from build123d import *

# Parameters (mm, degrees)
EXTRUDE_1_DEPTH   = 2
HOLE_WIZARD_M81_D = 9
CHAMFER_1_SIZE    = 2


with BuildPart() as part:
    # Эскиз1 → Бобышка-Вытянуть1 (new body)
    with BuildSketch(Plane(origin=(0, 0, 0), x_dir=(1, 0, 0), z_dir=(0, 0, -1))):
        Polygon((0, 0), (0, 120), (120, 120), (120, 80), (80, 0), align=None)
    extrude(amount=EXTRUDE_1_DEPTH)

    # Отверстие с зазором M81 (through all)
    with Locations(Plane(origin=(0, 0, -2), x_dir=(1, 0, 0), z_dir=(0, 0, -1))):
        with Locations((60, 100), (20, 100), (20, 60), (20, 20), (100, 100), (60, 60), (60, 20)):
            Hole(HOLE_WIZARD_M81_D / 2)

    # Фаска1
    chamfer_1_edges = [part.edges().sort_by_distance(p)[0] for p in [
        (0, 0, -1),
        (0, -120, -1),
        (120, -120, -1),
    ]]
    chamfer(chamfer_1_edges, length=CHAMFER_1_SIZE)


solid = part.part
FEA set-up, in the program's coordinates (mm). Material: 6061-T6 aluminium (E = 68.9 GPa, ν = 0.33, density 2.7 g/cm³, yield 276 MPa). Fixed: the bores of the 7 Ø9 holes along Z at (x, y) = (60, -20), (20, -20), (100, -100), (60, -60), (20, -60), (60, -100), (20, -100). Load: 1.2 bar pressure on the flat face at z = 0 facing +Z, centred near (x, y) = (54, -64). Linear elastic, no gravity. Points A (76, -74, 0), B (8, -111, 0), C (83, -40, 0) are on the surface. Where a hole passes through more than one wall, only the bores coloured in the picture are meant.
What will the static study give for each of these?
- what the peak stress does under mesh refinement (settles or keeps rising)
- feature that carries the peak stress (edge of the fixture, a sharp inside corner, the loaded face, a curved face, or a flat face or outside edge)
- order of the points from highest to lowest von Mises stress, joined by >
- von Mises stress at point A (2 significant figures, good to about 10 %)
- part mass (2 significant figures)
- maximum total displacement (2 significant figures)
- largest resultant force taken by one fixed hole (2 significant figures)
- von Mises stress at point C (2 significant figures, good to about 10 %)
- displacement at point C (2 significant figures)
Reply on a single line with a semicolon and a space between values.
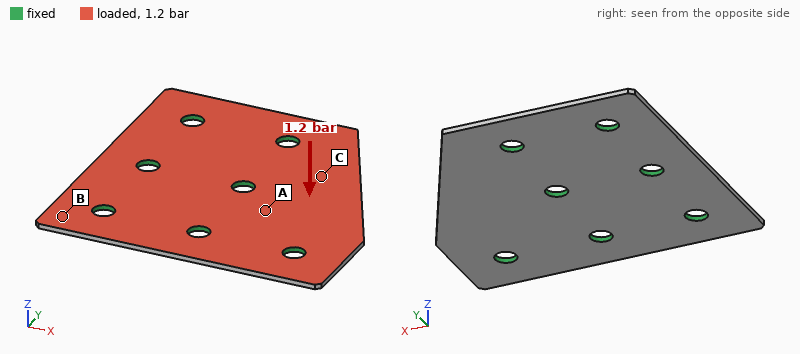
keeps rising; edge of the fixture; A > C > B; 30 MPa; 67 g; 0.43 mm; 260 N; 20 MPa; 0.20 mm
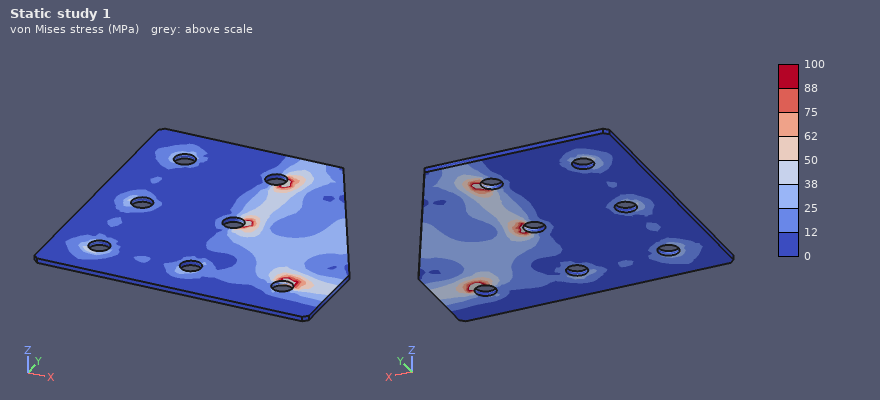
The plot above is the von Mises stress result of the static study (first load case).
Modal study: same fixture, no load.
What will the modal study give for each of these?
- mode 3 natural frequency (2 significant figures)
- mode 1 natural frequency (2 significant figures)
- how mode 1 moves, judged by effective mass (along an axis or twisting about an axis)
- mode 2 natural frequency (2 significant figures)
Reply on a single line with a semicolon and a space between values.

4000 Hz; 1600 Hz; along Z; 3000 Hz
